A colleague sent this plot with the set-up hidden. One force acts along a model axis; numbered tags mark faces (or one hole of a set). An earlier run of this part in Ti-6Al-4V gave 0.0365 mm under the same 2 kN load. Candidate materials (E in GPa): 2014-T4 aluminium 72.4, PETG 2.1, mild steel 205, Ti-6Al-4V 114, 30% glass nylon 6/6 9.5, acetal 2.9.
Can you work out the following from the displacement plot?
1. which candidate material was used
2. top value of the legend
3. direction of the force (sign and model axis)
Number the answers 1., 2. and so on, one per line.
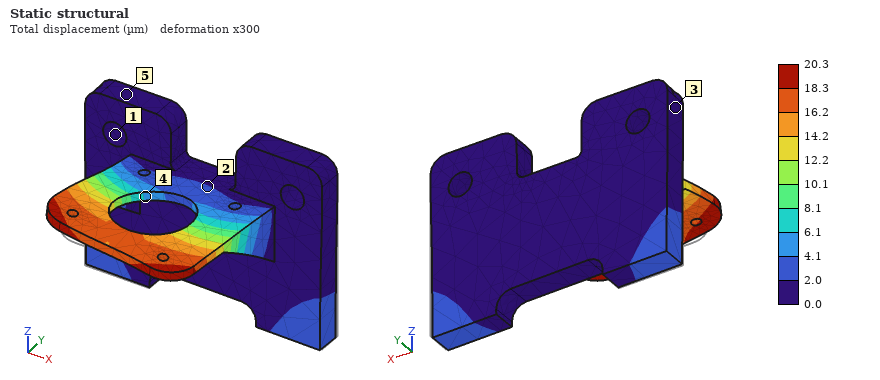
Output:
1. mild steel
2. 20.3 µm
3. -X
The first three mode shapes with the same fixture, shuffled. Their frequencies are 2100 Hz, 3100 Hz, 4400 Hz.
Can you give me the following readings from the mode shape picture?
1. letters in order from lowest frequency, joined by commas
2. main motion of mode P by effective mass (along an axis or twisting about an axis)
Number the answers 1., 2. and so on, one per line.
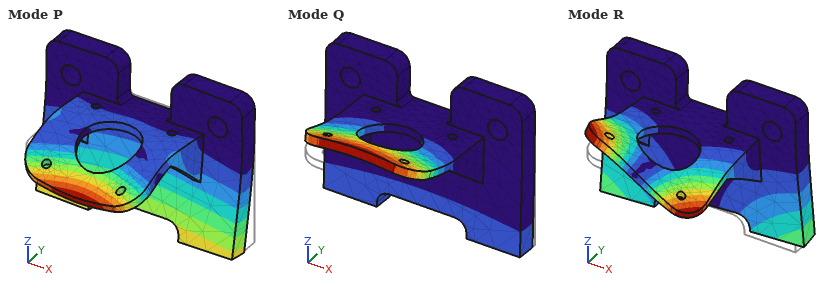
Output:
1. Q, P, R
2. along Y
